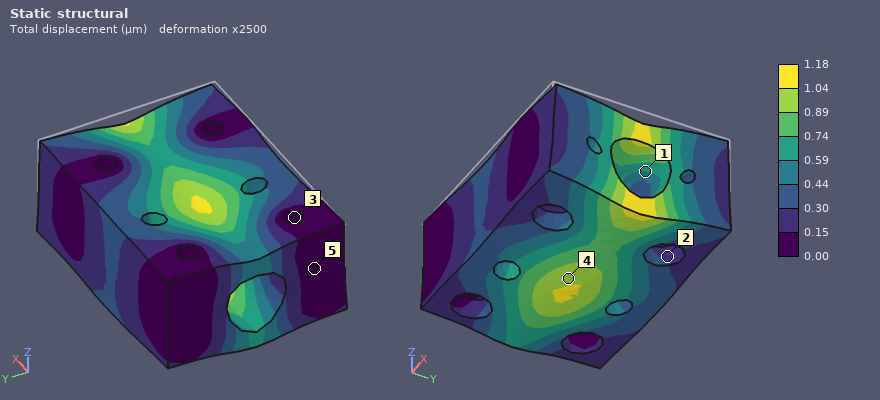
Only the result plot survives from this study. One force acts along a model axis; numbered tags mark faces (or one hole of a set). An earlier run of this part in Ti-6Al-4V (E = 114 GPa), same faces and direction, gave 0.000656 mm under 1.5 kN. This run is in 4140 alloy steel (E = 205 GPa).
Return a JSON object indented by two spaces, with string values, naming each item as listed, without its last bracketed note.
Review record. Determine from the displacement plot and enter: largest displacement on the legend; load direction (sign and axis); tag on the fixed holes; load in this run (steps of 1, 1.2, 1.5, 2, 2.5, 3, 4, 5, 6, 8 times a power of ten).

{
  "largest displacement on the legend": "1.18 µm",
  "load direction": "-Z",
  "tag on the fixed holes": "3",
  "load in this run": "5 kN"
}
